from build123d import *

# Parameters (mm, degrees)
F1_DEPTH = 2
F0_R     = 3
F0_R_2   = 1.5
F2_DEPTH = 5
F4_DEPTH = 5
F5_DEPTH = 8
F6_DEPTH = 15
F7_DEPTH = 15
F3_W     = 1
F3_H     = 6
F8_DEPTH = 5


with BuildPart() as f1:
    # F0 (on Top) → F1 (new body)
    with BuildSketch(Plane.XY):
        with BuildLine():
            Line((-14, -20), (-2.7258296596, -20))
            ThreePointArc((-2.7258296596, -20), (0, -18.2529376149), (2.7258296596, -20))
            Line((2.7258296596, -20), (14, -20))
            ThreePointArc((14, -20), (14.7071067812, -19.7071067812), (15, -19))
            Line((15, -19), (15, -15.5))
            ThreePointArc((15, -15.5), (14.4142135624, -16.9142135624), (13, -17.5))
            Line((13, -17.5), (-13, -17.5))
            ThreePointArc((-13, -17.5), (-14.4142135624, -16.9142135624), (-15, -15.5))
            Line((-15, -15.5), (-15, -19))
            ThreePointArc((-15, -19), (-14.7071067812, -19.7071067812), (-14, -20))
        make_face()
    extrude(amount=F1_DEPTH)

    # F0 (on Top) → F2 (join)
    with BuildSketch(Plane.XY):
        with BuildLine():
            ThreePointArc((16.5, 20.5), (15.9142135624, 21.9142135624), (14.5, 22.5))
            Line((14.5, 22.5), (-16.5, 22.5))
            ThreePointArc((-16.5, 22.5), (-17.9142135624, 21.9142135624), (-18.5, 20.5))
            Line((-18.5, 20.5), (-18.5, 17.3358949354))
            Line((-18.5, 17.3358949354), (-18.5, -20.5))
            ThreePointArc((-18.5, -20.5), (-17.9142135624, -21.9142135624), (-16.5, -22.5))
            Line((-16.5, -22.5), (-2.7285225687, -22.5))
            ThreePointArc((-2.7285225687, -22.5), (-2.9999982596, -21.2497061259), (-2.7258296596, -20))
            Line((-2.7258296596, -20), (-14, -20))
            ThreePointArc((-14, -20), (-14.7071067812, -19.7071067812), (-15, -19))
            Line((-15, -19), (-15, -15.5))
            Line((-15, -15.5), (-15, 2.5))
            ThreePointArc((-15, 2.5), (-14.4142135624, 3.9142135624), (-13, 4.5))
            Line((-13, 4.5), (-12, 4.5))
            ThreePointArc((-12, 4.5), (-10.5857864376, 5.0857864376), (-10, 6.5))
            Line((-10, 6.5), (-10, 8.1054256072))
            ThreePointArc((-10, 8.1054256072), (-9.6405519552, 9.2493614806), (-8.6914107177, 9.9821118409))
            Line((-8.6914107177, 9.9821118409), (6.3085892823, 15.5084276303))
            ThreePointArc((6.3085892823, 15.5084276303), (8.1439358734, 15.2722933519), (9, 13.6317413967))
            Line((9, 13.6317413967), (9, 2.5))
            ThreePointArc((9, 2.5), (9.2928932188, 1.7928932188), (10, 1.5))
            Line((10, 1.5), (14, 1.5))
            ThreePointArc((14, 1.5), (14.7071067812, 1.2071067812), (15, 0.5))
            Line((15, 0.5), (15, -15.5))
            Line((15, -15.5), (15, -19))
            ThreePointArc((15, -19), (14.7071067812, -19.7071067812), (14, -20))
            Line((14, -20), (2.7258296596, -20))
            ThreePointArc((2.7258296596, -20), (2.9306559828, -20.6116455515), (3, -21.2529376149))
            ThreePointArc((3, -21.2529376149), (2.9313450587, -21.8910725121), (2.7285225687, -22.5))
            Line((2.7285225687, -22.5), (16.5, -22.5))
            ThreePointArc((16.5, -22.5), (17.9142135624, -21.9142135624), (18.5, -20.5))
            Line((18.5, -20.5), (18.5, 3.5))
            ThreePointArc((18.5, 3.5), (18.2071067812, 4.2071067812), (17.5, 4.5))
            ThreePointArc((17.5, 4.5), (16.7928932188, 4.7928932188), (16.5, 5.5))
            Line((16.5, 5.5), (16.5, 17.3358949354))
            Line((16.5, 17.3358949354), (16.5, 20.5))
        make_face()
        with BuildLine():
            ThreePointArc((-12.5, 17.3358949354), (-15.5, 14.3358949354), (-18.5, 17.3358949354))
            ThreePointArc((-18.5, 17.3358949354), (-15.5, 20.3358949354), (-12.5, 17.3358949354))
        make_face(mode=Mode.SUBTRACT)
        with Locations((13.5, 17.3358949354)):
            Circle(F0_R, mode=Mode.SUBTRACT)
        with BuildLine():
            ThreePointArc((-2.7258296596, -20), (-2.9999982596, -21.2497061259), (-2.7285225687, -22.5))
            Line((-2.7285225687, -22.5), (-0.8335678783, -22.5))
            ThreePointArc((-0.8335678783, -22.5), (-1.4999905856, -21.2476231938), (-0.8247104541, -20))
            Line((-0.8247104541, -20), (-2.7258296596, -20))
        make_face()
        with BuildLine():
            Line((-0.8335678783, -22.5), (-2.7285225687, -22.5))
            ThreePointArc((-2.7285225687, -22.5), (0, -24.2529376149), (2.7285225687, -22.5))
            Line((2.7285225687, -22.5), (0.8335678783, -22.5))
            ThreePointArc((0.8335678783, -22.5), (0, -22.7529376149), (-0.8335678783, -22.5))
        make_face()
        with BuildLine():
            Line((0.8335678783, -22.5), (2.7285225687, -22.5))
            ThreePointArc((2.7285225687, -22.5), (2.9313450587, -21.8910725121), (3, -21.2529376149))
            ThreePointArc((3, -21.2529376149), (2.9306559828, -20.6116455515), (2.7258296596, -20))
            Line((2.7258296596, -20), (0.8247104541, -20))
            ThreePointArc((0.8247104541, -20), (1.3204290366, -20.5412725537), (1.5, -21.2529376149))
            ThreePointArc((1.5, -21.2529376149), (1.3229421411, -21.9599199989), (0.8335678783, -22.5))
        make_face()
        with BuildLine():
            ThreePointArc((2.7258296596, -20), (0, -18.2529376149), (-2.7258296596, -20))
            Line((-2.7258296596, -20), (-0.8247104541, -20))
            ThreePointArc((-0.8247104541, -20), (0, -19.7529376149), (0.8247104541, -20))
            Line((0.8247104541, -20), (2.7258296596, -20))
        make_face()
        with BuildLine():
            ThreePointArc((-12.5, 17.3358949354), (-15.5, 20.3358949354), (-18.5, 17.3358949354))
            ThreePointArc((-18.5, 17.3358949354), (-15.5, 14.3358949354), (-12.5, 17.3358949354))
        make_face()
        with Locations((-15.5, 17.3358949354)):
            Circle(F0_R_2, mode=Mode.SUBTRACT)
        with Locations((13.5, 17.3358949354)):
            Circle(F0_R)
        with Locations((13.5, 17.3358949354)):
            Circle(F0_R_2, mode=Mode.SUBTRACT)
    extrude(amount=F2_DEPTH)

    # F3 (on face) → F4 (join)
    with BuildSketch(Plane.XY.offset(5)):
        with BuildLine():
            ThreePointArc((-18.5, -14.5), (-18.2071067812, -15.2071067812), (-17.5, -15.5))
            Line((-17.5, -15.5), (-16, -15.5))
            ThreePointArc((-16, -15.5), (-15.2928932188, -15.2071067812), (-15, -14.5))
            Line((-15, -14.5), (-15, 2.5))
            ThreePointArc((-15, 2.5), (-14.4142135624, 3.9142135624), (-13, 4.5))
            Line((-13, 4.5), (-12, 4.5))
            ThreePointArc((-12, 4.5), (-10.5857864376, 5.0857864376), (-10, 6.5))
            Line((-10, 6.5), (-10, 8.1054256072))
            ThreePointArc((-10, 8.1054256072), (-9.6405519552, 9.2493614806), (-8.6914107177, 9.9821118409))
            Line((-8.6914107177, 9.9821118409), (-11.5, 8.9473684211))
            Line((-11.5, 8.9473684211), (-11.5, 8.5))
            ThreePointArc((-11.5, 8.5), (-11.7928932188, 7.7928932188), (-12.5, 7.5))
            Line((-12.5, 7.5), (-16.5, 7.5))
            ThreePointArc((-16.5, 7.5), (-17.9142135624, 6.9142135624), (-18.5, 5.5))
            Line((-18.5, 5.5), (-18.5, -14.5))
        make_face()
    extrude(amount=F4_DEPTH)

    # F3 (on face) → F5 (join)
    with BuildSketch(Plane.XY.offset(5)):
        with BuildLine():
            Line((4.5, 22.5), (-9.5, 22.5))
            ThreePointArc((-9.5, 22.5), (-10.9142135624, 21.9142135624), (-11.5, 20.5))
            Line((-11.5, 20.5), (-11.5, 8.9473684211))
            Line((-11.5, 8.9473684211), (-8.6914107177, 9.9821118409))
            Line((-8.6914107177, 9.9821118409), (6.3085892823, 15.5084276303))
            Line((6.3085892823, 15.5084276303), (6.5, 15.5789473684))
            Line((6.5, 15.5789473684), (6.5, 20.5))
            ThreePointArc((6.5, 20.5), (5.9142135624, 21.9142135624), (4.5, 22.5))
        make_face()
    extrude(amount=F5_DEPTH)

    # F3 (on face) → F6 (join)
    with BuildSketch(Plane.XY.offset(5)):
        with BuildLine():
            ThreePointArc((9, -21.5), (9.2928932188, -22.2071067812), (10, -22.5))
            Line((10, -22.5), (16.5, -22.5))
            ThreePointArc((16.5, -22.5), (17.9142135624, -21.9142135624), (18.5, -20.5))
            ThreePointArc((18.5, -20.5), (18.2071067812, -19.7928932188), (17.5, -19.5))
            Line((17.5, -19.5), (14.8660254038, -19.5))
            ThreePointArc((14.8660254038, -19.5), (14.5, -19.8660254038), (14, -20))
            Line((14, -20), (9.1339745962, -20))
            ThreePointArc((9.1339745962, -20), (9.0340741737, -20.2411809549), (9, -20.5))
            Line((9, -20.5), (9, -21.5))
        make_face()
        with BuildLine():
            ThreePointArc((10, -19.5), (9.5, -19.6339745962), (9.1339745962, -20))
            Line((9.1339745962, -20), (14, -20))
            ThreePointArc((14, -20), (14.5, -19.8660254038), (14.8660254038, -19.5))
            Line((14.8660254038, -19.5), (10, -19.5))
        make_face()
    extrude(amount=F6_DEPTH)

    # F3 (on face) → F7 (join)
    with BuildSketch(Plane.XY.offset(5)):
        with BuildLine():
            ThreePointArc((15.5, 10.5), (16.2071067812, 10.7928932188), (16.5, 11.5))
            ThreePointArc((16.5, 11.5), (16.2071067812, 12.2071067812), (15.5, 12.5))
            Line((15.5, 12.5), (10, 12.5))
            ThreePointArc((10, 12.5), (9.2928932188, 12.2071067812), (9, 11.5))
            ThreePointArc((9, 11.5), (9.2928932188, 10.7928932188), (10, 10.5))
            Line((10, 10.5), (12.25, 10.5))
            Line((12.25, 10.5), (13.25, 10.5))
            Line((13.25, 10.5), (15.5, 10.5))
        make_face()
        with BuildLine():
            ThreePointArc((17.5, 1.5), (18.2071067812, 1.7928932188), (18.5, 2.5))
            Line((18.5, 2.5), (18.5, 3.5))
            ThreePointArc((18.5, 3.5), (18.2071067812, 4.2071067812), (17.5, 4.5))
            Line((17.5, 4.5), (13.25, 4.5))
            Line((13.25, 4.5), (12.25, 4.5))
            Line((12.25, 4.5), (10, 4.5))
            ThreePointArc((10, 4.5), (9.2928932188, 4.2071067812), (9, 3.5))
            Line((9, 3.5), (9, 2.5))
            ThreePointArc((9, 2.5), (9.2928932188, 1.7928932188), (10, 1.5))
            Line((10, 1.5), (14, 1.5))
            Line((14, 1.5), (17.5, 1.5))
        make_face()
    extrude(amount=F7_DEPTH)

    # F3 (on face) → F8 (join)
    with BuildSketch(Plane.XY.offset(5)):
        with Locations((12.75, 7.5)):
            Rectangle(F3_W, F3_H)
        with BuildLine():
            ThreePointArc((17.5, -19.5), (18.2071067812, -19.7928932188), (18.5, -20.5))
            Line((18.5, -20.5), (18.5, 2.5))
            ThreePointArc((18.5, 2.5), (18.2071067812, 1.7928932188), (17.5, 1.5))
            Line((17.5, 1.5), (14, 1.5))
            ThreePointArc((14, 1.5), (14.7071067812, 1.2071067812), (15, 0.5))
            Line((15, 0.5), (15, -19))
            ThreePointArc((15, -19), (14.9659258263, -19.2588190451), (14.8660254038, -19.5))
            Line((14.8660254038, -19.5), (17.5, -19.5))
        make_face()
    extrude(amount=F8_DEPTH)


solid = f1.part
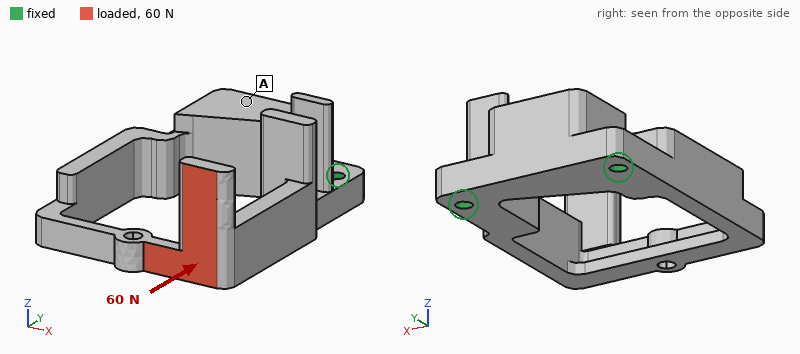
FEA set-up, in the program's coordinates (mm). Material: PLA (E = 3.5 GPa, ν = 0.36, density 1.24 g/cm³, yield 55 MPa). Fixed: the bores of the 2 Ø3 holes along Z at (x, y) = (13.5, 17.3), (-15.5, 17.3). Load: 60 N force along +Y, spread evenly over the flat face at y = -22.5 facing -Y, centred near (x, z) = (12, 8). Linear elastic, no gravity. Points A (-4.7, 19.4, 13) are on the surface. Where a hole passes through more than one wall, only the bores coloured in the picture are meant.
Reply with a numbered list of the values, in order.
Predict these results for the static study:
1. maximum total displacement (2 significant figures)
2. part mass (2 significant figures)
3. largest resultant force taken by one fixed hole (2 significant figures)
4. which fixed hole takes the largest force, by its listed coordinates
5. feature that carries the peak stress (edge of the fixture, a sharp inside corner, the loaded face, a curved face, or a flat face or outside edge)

1. 0.65 mm
2. 9.0 g
3. 53 N
4. (13.5, 17.3)
5. a curved face
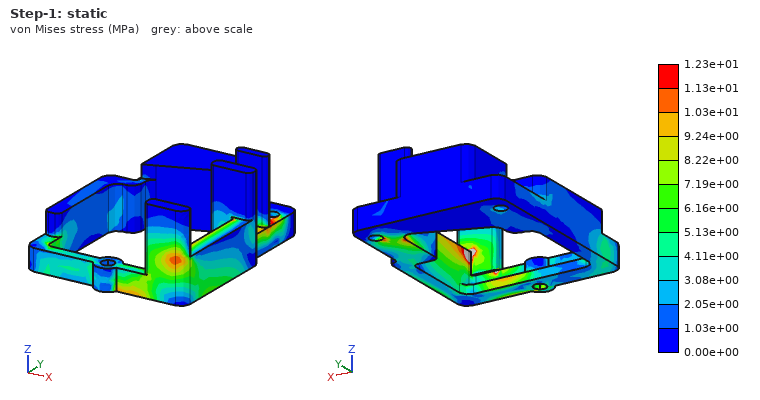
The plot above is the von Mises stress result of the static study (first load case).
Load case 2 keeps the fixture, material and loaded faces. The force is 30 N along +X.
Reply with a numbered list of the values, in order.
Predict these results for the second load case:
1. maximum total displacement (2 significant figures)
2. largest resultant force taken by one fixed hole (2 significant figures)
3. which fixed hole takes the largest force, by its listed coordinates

1. 0.64 mm
2. 39 N
3. (13.5, 17.3)
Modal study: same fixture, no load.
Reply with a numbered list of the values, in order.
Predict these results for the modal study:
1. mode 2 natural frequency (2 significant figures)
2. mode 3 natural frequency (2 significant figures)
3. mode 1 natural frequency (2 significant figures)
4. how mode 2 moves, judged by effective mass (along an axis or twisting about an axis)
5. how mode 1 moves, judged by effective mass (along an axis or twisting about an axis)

1. 970 Hz
2. 1300 Hz
3. 700 Hz
4. along X
5. along Z
